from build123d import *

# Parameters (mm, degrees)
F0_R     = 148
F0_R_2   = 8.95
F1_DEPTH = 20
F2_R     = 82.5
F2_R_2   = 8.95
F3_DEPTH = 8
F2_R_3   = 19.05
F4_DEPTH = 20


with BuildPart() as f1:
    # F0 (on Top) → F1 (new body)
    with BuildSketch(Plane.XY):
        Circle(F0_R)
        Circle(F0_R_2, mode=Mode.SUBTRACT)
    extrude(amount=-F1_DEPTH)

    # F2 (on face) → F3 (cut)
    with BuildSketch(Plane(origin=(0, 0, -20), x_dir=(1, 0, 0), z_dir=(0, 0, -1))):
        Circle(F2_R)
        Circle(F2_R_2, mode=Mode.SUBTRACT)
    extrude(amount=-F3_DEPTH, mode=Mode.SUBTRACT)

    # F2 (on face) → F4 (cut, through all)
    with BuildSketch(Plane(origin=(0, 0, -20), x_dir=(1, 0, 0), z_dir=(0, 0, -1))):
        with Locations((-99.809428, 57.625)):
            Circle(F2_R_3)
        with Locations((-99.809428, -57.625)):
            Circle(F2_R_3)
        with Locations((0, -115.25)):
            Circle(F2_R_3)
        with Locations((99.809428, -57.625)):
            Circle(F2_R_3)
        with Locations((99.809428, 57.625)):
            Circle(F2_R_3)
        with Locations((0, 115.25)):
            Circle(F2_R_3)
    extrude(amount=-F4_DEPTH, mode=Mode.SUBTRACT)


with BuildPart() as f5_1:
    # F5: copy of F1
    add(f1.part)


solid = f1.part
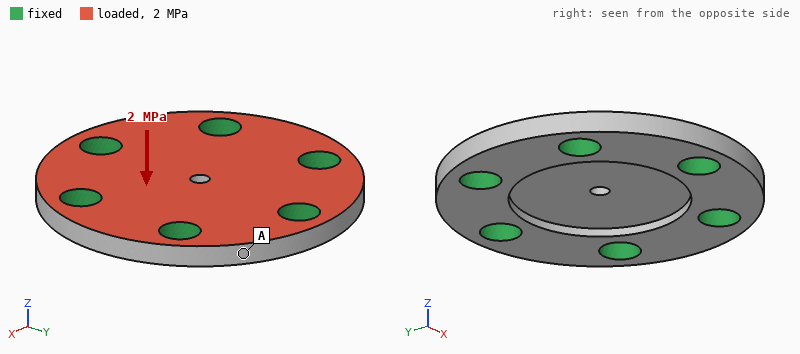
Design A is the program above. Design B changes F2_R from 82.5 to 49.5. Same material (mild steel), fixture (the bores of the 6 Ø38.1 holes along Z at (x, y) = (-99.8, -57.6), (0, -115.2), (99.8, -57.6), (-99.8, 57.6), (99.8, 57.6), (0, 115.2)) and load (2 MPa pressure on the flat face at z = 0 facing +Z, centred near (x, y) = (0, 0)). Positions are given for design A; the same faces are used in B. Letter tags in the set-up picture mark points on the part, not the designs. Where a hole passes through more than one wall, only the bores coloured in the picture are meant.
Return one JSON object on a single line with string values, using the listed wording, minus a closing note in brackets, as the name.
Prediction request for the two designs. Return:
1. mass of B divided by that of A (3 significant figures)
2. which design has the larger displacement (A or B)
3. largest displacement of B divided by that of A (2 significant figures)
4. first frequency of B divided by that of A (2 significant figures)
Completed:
{"mass of B divided by that of A": "1.10", "which design has the larger displacement": "A", "largest displacement of B divided by that of A": "0.55", "first frequency of B divided by that of A": "1.3"}
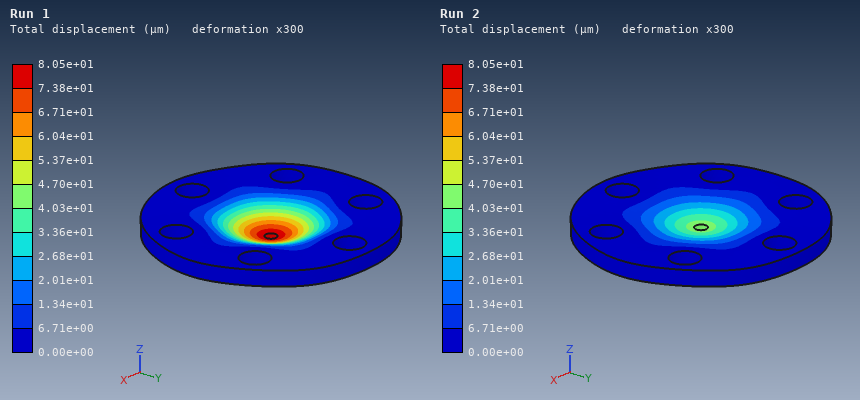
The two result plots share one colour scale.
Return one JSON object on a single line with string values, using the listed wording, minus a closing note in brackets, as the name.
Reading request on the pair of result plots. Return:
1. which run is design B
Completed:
{"which run is design B": "Run 2"}
